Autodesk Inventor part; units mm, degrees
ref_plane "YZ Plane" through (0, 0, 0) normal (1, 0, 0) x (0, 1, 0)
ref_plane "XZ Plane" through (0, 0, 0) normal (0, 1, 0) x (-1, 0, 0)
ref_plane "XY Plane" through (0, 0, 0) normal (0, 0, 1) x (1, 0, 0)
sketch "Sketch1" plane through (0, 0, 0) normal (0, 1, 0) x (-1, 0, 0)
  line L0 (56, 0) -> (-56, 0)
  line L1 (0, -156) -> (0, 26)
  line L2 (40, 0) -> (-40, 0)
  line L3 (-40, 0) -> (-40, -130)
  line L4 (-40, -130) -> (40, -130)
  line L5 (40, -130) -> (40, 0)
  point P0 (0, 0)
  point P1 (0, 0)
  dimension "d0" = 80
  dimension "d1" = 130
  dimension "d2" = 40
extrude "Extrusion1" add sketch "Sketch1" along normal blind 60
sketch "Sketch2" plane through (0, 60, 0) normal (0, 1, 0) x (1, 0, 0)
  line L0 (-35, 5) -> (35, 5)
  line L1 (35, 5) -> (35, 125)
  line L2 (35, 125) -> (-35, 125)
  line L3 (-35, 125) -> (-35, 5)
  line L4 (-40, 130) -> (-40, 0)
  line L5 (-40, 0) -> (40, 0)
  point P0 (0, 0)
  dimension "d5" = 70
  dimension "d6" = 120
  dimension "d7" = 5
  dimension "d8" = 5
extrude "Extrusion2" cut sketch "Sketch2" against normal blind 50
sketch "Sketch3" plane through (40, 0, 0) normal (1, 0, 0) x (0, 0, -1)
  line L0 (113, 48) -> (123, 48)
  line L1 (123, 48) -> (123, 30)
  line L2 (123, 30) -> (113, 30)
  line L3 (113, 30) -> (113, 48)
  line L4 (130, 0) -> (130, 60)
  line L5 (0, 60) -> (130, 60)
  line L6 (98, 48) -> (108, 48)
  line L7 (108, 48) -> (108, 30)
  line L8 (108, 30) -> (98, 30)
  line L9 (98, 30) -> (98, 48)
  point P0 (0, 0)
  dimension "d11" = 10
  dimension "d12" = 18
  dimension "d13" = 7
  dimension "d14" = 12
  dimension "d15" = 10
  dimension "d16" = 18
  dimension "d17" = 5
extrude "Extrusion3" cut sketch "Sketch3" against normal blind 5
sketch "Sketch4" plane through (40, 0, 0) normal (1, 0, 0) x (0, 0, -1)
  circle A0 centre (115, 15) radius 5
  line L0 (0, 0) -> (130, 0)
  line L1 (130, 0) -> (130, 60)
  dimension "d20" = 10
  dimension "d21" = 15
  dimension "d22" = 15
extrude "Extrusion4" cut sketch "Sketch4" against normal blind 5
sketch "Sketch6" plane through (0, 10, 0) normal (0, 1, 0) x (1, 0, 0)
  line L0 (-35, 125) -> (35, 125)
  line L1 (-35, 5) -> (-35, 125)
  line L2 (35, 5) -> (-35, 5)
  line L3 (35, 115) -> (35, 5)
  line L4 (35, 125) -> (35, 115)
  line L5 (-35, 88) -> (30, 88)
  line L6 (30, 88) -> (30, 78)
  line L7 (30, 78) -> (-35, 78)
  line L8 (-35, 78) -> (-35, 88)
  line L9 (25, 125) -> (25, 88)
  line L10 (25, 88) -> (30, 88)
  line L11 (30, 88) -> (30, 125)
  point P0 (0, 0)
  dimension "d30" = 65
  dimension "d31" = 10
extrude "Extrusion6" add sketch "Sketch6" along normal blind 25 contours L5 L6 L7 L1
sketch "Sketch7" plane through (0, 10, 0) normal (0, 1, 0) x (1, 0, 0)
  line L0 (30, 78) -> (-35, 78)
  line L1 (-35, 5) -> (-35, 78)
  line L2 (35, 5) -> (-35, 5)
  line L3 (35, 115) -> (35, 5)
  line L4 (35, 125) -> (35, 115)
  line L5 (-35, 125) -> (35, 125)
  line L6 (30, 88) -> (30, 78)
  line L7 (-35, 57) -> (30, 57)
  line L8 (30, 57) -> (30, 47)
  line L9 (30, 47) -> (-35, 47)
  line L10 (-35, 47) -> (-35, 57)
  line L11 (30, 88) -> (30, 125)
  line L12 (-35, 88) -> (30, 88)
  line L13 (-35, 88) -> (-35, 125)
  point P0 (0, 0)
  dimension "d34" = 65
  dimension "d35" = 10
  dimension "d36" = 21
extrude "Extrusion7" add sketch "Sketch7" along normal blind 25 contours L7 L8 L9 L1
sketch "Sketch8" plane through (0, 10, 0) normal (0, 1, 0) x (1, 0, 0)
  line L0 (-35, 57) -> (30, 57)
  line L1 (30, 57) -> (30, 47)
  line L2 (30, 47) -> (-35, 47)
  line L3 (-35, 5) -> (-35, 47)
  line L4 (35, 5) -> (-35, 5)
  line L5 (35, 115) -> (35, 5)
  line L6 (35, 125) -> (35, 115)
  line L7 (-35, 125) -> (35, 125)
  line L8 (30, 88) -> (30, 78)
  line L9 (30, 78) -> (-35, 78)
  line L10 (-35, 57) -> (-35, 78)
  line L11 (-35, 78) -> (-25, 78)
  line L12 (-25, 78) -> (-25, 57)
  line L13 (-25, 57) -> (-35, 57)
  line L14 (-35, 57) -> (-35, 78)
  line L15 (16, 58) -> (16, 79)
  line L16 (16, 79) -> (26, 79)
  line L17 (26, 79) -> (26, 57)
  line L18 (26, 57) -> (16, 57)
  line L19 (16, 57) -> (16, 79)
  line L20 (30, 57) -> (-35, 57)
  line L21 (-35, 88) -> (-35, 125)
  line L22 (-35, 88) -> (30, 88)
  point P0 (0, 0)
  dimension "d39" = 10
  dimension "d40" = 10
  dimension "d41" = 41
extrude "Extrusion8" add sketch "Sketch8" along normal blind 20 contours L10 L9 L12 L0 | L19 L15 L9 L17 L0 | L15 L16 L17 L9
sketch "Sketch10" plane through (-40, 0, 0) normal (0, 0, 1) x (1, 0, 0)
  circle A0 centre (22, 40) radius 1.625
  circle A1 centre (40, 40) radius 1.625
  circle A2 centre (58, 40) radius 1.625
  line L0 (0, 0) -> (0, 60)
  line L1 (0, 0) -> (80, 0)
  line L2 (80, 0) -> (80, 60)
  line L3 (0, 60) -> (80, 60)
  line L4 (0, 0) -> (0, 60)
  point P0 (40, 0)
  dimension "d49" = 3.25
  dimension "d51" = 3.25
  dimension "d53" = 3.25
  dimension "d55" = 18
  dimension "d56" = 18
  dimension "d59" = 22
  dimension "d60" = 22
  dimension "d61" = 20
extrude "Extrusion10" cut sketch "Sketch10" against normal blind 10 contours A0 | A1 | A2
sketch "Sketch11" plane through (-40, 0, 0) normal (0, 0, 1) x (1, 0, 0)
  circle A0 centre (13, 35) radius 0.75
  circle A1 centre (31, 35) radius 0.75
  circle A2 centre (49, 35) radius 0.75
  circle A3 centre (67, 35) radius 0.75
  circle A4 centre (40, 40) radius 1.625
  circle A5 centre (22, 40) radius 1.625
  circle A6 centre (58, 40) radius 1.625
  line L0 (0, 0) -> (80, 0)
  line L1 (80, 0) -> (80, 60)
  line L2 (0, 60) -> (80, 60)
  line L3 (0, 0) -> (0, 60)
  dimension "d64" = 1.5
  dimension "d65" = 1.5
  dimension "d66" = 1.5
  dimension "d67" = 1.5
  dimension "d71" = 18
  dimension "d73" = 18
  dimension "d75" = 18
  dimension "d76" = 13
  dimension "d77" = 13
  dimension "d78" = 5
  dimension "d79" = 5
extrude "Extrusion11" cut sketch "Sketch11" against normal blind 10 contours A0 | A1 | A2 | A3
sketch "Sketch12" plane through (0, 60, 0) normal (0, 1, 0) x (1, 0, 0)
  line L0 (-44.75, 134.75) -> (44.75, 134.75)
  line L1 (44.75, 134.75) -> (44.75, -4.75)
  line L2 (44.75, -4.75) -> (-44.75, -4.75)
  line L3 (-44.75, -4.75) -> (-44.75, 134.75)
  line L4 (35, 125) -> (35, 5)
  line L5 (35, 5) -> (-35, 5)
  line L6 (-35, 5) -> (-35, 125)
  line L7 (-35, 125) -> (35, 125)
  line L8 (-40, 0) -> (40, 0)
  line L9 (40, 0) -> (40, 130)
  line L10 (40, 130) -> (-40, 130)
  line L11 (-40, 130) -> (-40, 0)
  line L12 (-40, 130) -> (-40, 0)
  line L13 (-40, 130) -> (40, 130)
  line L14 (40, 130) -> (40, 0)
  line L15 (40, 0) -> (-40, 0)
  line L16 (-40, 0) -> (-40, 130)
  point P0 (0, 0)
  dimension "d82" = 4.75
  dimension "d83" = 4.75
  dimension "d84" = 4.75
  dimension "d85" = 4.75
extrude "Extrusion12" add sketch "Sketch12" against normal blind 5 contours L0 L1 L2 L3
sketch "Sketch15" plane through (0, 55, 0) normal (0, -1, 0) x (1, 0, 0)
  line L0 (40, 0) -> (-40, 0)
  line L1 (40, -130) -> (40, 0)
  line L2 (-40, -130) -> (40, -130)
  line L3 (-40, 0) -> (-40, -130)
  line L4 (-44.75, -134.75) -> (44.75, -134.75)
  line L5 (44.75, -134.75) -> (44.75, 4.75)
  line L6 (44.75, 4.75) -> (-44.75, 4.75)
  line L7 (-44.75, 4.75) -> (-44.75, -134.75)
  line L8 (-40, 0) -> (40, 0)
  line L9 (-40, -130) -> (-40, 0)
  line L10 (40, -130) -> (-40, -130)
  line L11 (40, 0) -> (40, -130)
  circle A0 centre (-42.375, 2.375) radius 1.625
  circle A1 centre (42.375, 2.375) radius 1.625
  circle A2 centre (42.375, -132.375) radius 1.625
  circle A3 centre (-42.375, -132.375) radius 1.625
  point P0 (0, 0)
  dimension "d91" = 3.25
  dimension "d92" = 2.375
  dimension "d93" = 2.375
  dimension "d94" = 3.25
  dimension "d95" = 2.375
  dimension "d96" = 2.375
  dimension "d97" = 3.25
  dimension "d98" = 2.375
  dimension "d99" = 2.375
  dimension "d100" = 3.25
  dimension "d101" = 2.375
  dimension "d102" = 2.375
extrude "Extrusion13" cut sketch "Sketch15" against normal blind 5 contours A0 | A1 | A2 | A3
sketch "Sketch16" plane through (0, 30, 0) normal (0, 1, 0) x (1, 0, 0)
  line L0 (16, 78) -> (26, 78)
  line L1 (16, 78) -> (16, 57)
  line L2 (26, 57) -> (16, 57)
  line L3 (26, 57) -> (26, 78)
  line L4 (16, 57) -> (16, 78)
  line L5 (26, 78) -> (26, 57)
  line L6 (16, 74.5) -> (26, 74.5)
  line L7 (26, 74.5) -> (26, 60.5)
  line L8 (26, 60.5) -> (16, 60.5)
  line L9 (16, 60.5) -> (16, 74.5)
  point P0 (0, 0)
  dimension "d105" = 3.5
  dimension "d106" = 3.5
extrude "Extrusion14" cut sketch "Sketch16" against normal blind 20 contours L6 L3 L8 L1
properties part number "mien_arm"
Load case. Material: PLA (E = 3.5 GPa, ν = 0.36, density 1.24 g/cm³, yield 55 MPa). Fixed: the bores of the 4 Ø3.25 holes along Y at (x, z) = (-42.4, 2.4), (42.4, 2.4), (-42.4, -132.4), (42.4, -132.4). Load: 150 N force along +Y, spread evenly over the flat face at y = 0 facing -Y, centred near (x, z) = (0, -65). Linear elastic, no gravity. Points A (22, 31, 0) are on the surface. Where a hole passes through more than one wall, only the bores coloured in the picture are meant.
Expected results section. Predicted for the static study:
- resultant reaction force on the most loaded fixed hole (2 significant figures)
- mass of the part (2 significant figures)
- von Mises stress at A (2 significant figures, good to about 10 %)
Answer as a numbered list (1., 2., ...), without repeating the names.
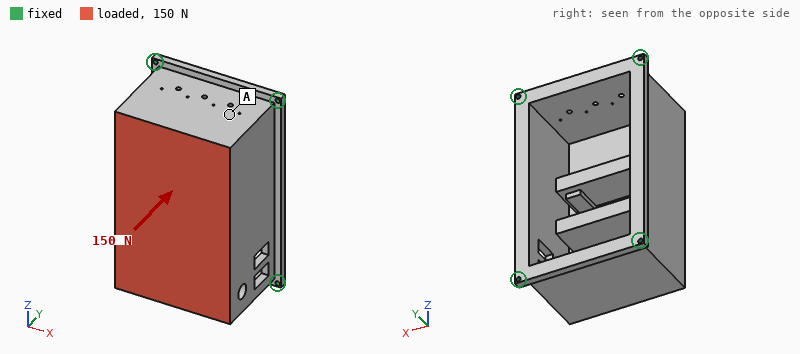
1. 48 N
2. 310 g
3. 0.14 MPa
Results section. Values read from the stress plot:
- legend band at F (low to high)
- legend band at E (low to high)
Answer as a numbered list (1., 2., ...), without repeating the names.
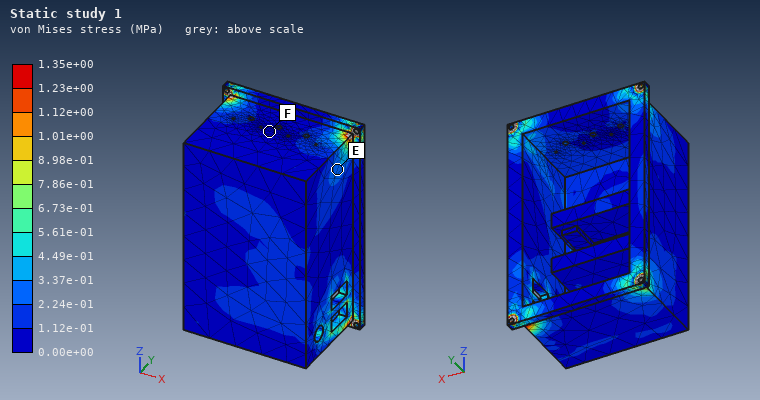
1. 0.00e+00 to 1.12e-01 MPa
2. 2.24e-01 to 3.37e-01 MPa
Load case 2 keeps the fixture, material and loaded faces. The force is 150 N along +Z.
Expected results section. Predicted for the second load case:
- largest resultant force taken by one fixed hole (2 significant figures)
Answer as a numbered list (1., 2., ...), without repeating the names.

1. 58 N
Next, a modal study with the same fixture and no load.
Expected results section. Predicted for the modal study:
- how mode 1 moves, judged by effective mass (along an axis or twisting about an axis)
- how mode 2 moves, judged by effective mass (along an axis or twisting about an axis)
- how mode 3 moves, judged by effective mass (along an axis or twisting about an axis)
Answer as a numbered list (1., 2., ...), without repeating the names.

1. along X
2. along Y
3. along Y
